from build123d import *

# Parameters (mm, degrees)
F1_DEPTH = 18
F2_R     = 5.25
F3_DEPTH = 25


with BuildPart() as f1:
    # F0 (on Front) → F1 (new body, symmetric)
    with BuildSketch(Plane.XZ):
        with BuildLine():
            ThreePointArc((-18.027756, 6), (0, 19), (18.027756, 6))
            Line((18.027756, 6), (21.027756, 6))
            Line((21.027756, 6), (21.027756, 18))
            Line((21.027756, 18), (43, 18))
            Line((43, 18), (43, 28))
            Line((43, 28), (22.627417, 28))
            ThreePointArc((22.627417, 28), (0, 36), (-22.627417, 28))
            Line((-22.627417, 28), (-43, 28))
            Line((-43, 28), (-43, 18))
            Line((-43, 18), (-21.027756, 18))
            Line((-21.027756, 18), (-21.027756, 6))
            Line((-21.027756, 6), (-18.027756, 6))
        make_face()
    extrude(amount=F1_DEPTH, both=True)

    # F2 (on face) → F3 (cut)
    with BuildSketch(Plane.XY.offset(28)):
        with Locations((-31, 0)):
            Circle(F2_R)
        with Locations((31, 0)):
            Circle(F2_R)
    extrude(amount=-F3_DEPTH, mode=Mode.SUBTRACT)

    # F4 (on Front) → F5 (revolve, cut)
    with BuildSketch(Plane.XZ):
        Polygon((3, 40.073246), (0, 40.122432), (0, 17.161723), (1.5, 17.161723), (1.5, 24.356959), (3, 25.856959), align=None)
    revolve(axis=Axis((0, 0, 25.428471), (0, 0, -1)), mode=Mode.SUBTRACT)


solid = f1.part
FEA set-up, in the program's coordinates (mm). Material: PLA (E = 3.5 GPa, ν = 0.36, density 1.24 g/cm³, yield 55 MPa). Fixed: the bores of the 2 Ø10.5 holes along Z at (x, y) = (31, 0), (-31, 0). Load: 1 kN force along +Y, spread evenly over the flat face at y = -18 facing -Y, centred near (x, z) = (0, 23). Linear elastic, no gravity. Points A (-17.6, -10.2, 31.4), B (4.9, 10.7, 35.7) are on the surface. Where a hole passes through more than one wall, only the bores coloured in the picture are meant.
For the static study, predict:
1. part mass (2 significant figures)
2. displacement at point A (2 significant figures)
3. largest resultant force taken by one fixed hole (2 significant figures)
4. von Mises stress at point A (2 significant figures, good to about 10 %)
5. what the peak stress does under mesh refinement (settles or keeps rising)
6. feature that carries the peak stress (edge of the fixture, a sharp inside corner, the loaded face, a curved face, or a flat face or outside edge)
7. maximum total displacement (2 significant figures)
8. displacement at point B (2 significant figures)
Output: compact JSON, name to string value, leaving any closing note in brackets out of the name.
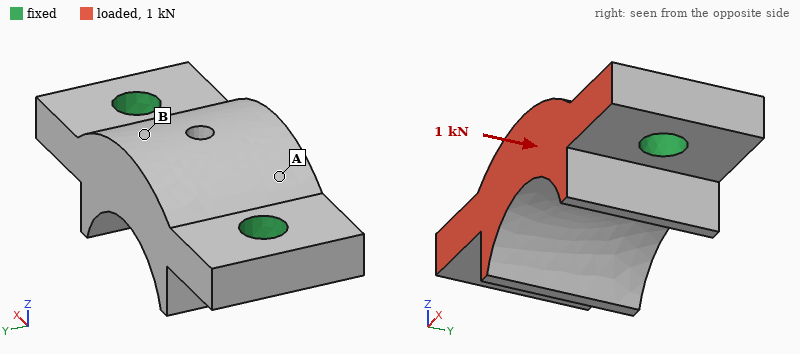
{"part mass": "54 g", "displacement at point A": "16 µm", "largest resultant force taken by one fixed hole": "500 N", "von Mises stress at point A": "1.4 MPa", "what the peak stress does under mesh refinement": "keeps rising", "feature that carries the peak stress": "edge of the fixture", "maximum total displacement": "27 µm", "displacement at point B": "20 µm"}
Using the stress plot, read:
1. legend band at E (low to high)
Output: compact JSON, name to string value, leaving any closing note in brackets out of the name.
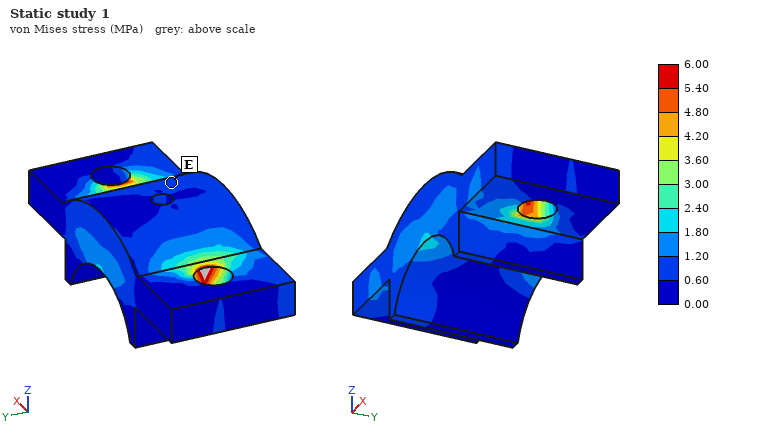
{"legend band at E": "0.60 to 1.20 MPa"}
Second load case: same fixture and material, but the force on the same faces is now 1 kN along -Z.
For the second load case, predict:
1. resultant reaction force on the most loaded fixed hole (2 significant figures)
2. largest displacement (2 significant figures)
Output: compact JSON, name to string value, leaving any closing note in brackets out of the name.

{"resultant reaction force on the most loaded fixed hole": "510 N", "largest displacement": "0.15 mm"}
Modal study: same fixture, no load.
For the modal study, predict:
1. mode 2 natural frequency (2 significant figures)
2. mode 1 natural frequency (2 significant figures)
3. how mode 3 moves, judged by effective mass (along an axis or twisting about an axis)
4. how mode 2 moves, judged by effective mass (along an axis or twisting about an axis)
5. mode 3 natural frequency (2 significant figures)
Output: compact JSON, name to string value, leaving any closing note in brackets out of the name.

{"mode 2 natural frequency": "4100 Hz", "mode 1 natural frequency": "3600 Hz", "how mode 3 moves, judged by effective mass": "along Y", "how mode 2 moves, judged by effective mass": "along Z", "mode 3 natural frequency": "5400 Hz"}
